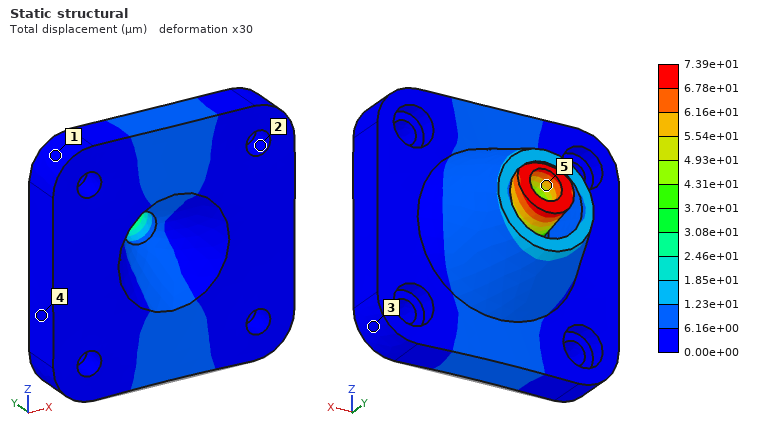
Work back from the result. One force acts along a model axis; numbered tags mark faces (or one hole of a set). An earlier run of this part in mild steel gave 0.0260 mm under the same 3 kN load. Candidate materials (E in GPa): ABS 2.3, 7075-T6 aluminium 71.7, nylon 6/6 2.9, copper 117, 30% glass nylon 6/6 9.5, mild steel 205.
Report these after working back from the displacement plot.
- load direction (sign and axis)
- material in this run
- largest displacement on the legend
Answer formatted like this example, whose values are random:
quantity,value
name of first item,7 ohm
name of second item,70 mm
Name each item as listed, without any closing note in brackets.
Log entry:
quantity,value
load direction,+Z
material in this run,7075-T6 aluminium
largest displacement on the legend,7.39e+01 µm
